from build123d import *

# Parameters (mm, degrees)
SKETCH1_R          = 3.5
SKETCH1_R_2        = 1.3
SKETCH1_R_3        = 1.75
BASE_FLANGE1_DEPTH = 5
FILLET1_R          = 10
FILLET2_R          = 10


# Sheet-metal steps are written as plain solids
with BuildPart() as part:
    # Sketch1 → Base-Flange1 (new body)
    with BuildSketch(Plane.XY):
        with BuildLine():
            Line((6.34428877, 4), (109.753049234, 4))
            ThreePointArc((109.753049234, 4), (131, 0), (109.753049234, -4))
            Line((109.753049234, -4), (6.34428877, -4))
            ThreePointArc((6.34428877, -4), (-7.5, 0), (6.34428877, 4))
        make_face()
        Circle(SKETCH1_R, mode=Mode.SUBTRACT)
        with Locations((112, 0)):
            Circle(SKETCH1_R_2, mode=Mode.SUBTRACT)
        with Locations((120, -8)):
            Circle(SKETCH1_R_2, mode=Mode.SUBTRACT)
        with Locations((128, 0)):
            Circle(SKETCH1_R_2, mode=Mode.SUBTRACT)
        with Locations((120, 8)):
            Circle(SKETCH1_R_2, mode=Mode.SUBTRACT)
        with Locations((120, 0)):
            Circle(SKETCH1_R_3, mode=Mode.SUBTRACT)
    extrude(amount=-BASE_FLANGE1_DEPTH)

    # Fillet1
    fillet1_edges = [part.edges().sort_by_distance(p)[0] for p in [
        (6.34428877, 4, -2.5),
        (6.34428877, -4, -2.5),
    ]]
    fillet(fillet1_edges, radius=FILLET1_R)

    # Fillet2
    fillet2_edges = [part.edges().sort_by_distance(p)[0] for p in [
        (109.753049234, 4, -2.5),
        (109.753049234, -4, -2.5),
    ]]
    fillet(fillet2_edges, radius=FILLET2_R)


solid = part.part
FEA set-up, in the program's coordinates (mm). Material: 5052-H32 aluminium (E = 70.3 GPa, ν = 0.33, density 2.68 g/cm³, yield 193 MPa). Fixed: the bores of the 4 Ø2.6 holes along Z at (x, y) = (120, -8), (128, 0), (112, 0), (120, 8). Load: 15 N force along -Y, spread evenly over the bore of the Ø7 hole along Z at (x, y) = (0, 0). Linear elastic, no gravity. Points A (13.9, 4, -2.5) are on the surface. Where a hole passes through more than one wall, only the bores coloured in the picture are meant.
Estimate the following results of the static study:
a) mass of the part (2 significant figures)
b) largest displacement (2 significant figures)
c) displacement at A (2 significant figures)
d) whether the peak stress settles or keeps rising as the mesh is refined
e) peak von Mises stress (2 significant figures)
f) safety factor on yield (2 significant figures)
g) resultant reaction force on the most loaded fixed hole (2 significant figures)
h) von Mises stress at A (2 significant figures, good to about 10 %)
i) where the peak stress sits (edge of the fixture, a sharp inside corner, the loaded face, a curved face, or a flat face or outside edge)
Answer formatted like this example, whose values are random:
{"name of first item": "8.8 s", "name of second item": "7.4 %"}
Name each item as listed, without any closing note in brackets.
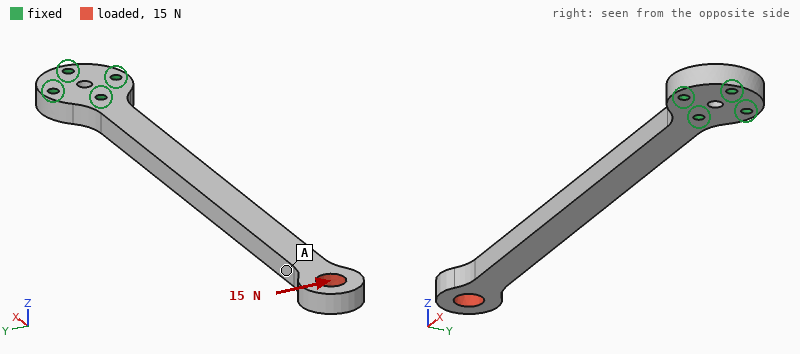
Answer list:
{"mass of the part": "18 g", "largest displacement": "0.49 mm", "displacement at A": "0.36 mm", "whether the peak stress settles or keeps rising as the mesh is refined": "settles", "peak von Mises stress": "32 MPa", "safety factor on yield": "6.1", "resultant reaction force on the most loaded fixed hole": "87 N", "von Mises stress at A": "4.0 MPa", "where the peak stress sits": "a curved face"}
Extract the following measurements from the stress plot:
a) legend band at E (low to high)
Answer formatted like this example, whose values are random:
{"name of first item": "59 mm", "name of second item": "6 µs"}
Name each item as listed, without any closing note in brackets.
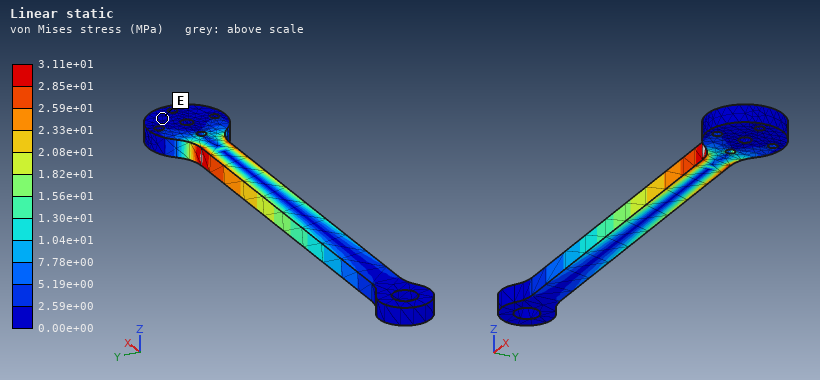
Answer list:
{"legend band at E": "0.00e+00 to 2.59e+00 MPa"}
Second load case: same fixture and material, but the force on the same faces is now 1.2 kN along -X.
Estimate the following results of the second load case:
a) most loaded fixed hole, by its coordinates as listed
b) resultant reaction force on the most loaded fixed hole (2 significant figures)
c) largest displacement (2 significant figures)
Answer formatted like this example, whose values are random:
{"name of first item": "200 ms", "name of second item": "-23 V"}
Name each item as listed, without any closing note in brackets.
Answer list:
{"most loaded fixed hole, by its coordinates as listed": "(112, 0)", "resultant reaction force on the most loaded fixed hole": "900 N", "largest displacement": "52 µm"}
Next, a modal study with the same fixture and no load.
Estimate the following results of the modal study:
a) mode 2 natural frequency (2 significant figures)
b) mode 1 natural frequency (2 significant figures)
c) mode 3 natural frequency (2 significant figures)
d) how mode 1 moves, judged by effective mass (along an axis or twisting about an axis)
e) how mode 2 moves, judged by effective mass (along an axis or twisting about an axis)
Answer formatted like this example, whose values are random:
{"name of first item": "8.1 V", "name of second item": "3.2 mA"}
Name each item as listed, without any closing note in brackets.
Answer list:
{"mode 2 natural frequency": "460 Hz", "mode 1 natural frequency": "280 Hz", "mode 3 natural frequency": "1800 Hz", "how mode 1 moves, judged by effective mass": "along Z", "how mode 2 moves, judged by effective mass": "along Y"}
